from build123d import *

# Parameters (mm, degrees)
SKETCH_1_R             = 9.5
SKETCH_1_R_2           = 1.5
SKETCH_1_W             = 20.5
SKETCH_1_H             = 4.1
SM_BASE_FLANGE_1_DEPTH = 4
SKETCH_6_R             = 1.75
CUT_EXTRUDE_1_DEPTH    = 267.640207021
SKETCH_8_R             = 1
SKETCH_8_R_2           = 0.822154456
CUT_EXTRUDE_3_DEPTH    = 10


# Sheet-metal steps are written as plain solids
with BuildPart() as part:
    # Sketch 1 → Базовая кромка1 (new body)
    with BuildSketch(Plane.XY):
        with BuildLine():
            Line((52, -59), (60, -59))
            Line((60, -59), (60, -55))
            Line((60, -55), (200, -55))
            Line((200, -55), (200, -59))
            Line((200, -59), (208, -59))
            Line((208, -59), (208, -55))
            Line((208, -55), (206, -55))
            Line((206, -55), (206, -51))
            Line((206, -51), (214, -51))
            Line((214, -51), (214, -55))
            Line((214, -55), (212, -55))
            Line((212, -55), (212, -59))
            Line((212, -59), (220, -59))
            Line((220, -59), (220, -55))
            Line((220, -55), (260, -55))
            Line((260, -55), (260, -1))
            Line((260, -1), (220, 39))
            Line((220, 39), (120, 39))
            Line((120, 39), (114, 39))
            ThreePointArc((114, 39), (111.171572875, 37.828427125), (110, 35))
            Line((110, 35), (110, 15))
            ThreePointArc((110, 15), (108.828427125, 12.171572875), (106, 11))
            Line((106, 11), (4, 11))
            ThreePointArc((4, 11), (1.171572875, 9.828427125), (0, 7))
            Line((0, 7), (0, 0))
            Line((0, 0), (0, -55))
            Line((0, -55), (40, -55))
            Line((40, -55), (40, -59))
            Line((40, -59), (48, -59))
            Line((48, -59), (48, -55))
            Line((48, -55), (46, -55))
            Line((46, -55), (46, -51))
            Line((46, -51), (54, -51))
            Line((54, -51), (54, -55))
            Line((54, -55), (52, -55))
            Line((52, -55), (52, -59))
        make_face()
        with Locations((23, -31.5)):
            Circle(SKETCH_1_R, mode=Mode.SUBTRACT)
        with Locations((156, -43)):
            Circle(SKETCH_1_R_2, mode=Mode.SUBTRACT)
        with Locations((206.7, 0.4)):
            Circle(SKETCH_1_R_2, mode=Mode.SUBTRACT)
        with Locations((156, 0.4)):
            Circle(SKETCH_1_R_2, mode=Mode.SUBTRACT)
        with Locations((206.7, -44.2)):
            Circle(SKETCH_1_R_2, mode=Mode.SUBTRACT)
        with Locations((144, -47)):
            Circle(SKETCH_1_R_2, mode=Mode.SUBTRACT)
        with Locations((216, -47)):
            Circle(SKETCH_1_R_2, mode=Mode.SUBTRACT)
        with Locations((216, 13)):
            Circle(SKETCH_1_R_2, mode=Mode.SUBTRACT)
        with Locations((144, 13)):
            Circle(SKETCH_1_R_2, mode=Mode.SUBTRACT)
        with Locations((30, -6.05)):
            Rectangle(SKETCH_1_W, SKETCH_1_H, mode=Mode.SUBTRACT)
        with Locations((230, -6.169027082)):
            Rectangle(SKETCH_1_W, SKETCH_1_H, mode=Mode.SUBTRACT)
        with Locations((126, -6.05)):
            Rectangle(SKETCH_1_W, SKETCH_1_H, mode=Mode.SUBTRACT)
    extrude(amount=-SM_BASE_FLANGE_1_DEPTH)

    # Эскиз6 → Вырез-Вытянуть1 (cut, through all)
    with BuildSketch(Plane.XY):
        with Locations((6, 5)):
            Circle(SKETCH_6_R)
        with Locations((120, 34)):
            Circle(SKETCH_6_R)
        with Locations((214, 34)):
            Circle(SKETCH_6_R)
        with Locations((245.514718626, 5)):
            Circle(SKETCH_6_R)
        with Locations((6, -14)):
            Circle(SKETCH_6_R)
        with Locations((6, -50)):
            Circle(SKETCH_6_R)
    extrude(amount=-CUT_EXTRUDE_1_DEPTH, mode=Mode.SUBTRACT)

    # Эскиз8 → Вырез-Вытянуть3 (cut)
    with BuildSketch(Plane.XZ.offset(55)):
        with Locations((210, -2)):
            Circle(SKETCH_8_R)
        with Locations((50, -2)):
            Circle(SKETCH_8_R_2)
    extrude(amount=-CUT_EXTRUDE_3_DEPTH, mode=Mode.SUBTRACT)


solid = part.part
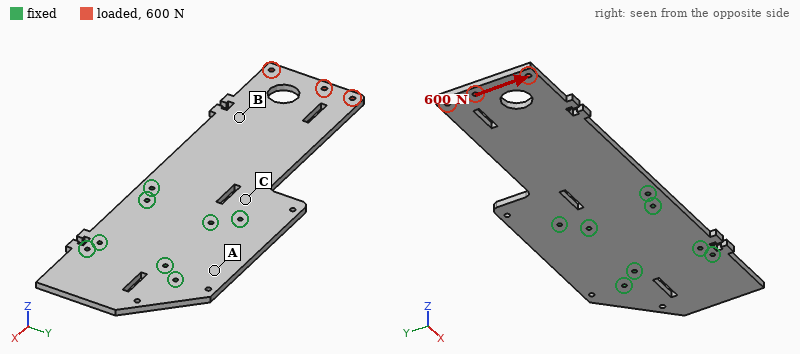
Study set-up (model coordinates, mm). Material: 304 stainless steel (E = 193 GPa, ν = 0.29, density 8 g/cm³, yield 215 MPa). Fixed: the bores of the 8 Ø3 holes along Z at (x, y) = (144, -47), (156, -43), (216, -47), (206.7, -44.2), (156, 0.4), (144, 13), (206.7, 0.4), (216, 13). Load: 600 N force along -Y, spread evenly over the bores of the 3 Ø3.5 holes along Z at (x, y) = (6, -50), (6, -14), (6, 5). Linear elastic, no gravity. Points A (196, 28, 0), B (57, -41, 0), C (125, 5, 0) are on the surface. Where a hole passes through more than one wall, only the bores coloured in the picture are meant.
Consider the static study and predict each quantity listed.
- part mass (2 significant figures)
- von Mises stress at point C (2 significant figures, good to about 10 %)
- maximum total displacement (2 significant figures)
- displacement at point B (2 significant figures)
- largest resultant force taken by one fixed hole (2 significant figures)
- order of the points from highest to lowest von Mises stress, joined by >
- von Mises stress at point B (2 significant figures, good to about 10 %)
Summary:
640 g
14 MPa
35 µm
15 µm
990 N
C > B > A
7.1 MPa
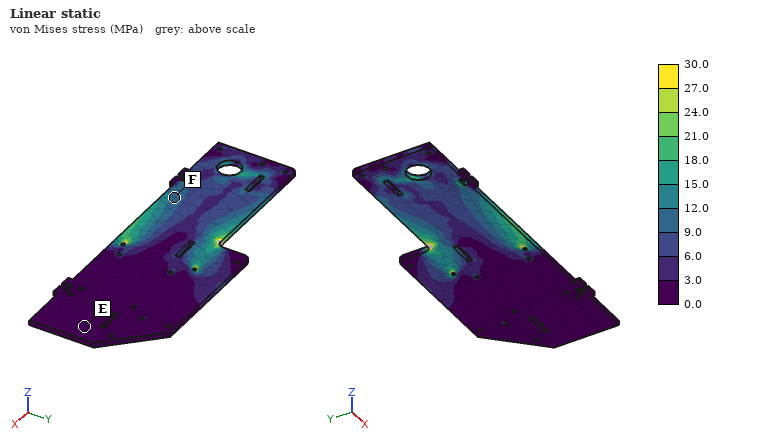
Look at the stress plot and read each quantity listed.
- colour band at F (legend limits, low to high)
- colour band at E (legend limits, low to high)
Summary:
9.0 to 12.0 MPa
0.0 to 3.0 MPa
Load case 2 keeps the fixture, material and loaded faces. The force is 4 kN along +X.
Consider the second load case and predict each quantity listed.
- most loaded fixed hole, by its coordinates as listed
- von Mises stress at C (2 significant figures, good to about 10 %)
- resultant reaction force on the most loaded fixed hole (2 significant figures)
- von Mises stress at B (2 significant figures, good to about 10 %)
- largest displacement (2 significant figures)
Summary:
(144, -47)
15 MPa
1.3 kN
15 MPa
14 µm
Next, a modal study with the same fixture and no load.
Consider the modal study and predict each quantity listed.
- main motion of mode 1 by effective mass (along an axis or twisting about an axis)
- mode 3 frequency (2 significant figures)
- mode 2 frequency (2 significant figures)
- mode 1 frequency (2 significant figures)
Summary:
along Z
940 Hz
730 Hz
160 Hz
